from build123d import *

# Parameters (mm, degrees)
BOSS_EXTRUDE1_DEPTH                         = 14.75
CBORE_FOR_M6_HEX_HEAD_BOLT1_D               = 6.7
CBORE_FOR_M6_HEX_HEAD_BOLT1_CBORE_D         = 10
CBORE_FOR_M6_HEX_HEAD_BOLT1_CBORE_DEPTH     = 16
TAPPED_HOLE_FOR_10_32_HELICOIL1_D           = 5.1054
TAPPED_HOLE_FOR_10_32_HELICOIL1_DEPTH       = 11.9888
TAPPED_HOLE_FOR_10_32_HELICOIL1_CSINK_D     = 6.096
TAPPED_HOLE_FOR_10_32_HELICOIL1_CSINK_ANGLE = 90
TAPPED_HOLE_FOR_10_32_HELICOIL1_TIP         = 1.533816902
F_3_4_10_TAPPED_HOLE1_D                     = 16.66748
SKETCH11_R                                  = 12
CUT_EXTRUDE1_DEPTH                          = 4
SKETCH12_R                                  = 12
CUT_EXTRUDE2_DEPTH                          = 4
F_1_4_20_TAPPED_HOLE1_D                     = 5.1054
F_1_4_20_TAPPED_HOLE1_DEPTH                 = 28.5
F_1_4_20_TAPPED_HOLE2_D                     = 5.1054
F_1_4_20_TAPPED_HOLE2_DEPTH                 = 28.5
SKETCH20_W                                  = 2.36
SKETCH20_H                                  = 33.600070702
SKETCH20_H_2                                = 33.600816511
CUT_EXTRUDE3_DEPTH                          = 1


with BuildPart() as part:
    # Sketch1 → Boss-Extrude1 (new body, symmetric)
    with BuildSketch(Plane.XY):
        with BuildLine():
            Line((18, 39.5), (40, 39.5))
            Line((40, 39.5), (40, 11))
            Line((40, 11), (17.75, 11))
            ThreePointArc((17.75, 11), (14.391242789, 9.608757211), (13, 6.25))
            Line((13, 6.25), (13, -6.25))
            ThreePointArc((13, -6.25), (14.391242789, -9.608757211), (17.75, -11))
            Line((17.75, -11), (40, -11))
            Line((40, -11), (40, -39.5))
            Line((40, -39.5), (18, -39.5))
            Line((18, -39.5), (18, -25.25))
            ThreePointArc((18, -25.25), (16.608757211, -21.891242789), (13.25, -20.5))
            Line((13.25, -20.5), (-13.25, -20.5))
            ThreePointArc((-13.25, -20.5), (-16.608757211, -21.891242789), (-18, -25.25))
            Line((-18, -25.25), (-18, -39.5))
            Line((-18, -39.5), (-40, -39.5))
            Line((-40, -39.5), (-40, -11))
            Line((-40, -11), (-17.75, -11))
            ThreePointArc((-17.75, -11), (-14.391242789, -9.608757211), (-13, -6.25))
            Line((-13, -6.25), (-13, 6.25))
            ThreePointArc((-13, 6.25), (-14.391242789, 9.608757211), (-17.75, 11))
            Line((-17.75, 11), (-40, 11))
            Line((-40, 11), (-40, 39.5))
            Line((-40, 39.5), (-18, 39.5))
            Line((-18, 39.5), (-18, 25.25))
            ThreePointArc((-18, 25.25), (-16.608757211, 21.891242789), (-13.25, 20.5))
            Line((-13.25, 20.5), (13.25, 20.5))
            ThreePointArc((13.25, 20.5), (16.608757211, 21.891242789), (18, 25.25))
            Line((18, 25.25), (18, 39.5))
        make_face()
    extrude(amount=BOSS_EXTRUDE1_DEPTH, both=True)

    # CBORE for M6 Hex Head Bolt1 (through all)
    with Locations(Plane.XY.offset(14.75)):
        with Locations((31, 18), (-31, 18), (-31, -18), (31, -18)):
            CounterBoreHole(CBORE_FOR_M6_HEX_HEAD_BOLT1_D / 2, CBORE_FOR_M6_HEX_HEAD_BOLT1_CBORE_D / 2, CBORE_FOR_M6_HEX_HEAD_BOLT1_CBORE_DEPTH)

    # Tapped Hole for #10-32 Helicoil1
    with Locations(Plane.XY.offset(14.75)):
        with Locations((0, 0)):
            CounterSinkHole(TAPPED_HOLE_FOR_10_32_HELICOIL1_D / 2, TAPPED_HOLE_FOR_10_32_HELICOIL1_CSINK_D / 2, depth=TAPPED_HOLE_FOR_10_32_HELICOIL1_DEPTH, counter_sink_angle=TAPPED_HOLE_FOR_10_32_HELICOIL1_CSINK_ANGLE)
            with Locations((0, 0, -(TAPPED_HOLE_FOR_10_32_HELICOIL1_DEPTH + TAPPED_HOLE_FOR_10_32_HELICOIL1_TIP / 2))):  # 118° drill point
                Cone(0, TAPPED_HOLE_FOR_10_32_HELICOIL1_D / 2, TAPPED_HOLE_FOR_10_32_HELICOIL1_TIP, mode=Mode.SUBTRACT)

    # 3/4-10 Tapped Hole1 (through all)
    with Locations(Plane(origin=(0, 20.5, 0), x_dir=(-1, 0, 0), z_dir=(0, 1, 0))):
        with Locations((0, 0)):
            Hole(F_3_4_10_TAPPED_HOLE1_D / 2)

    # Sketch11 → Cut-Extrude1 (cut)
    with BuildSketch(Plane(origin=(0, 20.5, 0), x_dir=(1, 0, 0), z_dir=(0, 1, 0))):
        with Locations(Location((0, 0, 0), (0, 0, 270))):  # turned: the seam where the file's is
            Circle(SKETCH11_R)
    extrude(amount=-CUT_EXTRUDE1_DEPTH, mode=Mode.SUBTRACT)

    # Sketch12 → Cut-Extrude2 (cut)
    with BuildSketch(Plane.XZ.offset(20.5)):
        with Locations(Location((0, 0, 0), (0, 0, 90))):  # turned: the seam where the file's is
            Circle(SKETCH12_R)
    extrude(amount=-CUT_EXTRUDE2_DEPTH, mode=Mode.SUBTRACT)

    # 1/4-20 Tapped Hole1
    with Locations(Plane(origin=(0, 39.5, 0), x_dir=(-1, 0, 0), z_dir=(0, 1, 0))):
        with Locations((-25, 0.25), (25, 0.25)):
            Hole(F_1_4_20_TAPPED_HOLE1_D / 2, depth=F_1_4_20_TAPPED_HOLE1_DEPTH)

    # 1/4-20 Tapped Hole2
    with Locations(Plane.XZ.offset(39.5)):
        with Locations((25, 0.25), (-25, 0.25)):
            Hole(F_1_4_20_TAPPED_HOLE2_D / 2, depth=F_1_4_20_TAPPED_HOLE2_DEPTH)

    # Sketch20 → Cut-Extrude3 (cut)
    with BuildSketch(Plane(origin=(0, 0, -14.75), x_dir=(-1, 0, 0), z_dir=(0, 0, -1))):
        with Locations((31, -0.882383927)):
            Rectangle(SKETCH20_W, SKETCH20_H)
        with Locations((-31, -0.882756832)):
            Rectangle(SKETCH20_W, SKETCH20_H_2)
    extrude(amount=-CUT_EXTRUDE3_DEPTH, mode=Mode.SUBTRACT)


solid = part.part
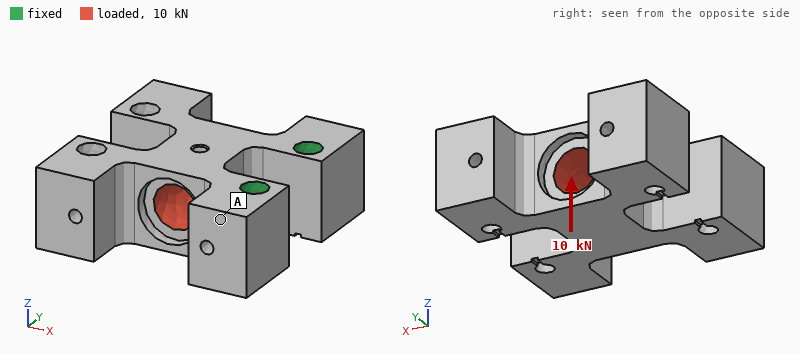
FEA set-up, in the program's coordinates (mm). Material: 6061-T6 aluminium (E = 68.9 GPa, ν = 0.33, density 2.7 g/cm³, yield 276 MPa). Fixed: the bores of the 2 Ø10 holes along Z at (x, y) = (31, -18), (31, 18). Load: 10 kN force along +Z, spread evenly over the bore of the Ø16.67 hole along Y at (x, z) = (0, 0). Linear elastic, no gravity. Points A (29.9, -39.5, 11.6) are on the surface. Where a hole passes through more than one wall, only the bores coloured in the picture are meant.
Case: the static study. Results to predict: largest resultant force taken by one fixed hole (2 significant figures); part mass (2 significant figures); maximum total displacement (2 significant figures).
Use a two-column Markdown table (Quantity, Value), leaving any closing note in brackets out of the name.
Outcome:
| Quantity | Value |
|---|---|
| largest resultant force taken by one fixed hole | 5.0 kN |
| part mass | 250 g |
| maximum total displacement | 0.20 mm |
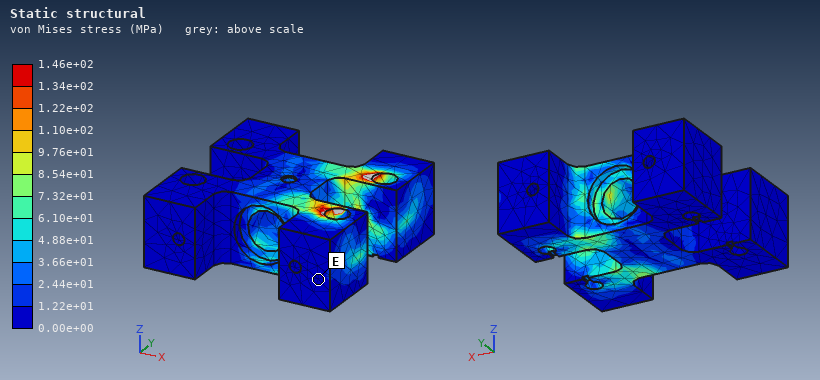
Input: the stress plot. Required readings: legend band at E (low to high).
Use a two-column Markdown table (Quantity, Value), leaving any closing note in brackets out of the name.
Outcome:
| Quantity | Value |
|---|---|
| legend band at E | 0.00e+00 to 1.22e+01 MPa |
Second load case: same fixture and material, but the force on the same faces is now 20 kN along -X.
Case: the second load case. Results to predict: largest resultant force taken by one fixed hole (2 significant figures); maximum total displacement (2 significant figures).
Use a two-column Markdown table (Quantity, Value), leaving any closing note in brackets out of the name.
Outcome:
| Quantity | Value |
|---|---|
| largest resultant force taken by one fixed hole | 10 kN |
| maximum total displacement | 68 µm |
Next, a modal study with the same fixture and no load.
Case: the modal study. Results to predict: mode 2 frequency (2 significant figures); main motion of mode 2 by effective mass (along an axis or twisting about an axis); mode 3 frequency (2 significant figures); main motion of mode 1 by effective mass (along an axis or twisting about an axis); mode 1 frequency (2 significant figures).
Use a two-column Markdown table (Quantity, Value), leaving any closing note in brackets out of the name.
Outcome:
| Quantity | Value |
|---|---|
| mode 2 frequency | 2700 Hz |
| main motion of mode 2 by effective mass | along Y |
| mode 3 frequency | 3300 Hz |
| main motion of mode 1 by effective mass | along Z |
| mode 1 frequency | 2400 Hz |
